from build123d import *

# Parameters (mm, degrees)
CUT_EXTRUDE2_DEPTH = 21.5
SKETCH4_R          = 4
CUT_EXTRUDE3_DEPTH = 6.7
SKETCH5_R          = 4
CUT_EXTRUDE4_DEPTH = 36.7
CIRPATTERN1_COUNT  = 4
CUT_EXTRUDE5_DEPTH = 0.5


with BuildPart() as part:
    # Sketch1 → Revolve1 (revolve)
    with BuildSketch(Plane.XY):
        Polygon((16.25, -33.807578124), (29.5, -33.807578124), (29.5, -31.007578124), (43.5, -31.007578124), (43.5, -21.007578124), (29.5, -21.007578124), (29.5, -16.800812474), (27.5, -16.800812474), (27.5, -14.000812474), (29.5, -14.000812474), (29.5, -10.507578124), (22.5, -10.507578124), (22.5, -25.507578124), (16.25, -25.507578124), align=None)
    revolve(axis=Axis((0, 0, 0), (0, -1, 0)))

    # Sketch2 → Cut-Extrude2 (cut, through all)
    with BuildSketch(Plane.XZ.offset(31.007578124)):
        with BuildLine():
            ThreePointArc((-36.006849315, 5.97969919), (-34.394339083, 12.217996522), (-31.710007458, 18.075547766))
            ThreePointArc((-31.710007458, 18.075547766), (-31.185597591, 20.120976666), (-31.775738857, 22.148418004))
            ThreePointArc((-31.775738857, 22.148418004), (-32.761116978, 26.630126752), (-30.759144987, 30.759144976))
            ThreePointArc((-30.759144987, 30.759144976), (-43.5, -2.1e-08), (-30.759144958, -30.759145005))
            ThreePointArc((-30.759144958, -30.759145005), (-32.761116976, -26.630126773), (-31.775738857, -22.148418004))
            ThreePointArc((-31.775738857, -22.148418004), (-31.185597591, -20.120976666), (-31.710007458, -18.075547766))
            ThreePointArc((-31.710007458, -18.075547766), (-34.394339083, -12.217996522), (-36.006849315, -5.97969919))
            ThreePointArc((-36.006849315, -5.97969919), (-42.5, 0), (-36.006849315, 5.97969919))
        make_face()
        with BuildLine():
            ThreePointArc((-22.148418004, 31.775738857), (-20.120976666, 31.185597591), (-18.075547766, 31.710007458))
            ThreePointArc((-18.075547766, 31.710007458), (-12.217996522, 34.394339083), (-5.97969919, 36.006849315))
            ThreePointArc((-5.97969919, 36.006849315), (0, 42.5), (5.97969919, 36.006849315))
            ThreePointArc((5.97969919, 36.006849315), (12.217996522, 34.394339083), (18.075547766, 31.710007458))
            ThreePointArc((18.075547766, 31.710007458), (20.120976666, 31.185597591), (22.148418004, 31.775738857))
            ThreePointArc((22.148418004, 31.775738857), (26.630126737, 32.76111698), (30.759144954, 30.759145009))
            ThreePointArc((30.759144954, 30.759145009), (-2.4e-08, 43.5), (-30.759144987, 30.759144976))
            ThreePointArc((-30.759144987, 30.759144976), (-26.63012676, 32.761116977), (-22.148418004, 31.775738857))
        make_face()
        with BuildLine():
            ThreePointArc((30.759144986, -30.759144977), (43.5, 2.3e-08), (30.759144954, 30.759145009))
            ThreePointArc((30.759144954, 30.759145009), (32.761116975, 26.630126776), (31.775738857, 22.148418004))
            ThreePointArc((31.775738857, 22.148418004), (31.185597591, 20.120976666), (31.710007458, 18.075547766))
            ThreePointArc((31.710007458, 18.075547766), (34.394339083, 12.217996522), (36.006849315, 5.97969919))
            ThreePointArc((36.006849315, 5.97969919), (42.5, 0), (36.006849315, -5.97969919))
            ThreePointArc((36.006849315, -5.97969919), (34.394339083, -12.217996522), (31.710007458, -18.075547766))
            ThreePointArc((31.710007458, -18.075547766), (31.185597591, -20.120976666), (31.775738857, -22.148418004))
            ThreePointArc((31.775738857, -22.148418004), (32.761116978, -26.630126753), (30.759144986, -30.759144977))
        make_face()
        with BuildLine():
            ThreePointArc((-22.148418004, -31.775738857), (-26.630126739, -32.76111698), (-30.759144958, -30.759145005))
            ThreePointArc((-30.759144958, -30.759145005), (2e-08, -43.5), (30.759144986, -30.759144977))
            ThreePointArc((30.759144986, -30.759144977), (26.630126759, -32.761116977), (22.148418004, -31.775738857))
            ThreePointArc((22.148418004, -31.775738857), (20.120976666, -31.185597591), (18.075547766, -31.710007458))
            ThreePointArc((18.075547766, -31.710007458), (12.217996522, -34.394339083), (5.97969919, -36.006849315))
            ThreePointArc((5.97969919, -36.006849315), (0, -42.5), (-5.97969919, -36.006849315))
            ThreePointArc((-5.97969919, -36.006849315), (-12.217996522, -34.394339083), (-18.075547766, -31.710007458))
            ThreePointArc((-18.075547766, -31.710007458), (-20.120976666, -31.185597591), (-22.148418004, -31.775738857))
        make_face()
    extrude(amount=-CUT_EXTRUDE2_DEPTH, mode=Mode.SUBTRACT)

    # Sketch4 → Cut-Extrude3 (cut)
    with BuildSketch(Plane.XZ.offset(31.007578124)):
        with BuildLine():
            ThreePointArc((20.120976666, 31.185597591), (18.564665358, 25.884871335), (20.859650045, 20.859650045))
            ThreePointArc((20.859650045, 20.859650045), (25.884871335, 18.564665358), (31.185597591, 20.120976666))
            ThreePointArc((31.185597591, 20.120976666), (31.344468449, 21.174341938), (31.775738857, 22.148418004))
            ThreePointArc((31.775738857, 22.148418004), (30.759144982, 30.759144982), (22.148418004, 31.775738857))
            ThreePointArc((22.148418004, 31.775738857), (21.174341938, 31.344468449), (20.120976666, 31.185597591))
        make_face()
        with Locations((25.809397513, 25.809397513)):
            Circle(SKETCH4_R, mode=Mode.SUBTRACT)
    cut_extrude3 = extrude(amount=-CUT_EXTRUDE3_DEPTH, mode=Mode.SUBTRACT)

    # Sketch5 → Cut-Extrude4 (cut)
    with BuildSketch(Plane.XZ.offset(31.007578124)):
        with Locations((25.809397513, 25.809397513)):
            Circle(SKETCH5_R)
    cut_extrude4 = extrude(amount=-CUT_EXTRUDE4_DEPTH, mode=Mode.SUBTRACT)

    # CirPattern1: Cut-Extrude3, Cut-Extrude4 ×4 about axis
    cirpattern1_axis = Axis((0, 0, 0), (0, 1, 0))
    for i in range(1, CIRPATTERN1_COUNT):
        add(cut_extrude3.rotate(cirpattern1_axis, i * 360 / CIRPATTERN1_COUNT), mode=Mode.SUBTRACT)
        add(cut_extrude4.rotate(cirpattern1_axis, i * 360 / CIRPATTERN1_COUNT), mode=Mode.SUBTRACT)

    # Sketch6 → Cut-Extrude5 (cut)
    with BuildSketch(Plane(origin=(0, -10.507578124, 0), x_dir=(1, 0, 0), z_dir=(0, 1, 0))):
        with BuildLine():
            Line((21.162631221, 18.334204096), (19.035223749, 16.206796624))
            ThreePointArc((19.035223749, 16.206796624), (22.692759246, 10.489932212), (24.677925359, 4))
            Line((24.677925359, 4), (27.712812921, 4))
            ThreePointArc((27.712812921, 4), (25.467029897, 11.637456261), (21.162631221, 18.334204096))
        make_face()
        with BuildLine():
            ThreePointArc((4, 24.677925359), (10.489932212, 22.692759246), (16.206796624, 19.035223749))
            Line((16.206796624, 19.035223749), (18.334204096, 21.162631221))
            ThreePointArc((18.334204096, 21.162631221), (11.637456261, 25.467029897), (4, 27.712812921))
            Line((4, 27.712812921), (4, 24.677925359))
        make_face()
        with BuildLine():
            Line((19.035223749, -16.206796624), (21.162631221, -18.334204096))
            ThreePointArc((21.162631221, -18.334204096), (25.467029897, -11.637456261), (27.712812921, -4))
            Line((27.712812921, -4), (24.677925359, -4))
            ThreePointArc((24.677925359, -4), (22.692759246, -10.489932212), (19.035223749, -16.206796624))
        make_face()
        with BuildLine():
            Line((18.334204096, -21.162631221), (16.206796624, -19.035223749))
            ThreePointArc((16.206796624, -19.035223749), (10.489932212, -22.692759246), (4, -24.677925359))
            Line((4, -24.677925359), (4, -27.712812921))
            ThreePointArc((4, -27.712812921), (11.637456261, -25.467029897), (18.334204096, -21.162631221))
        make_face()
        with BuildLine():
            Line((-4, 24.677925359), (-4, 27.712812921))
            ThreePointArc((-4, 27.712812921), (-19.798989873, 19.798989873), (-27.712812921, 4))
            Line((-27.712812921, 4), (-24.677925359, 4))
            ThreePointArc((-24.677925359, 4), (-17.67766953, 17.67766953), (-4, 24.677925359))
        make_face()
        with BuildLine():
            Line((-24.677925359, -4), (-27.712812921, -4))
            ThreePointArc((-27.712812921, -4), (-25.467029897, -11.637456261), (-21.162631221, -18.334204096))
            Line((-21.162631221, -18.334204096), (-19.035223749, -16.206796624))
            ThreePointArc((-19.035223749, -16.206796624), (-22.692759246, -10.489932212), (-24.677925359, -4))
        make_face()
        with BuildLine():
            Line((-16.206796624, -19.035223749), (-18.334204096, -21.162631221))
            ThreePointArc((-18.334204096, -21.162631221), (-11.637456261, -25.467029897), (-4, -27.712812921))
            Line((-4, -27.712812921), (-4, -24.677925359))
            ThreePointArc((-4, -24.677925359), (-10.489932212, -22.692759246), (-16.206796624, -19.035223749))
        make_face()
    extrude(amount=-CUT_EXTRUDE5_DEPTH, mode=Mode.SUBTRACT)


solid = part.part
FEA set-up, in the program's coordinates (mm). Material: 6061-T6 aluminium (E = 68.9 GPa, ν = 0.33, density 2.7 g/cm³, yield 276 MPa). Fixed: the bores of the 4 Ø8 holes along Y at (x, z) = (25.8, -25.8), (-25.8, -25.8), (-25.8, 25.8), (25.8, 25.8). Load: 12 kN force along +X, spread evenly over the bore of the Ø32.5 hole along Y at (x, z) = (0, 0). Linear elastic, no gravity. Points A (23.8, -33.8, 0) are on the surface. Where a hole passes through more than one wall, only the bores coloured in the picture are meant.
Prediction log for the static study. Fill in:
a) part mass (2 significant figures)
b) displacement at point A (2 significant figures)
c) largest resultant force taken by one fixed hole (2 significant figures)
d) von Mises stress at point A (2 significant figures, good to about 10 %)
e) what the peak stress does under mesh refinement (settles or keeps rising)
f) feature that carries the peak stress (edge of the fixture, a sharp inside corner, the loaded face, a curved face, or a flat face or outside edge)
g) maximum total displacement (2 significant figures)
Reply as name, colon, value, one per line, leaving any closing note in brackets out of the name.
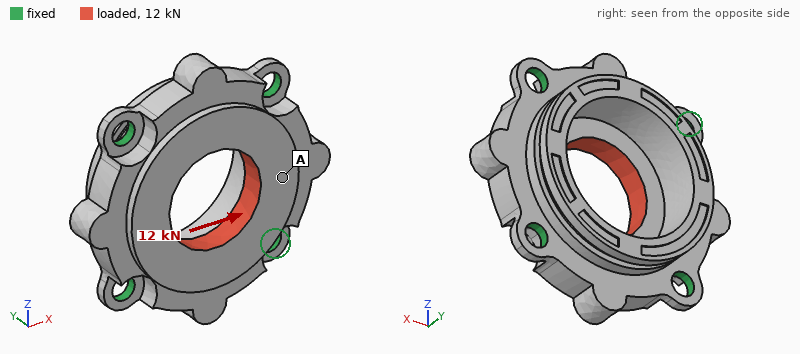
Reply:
part mass: 130 g
displacement at point A: 19 µm
largest resultant force taken by one fixed hole: 3.2 kN
von Mises stress at point A: 15 MPa
what the peak stress does under mesh refinement: keeps rising
feature that carries the peak stress: edge of the fixture
maximum total displacement: 21 µm
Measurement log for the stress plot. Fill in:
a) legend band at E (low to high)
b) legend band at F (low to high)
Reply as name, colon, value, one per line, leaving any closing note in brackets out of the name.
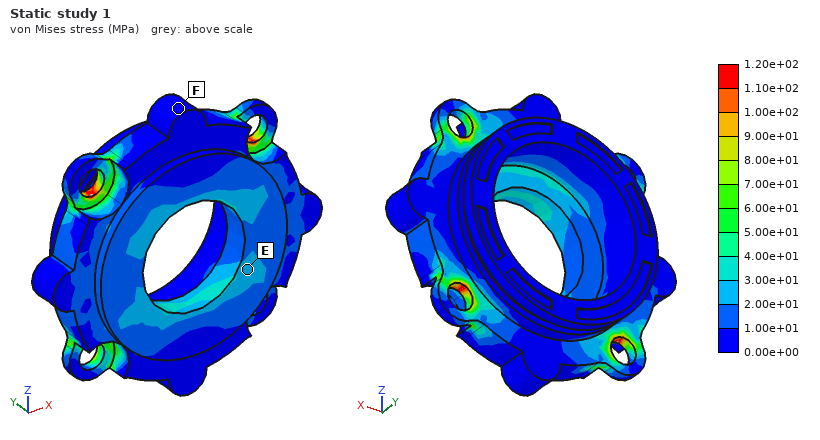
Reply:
legend band at E: 2.00e+01 to 3.00e+01 MPa
legend band at F: 0.00e+00 to 1.00e+01 MPa
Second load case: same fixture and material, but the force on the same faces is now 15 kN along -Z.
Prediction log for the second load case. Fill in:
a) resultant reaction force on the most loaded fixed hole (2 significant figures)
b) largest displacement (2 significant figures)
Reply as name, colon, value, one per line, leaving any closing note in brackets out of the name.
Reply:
resultant reaction force on the most loaded fixed hole: 4.0 kN
largest displacement: 26 µm
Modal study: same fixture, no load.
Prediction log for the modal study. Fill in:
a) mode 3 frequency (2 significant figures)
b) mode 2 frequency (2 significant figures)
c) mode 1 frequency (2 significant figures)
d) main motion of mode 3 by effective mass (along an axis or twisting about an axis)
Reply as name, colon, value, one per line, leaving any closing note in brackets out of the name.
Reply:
mode 3 frequency: 12 kHz
mode 2 frequency: 11 kHz
mode 1 frequency: 11 kHz
main motion of mode 3 by effective mass: twisting about X
